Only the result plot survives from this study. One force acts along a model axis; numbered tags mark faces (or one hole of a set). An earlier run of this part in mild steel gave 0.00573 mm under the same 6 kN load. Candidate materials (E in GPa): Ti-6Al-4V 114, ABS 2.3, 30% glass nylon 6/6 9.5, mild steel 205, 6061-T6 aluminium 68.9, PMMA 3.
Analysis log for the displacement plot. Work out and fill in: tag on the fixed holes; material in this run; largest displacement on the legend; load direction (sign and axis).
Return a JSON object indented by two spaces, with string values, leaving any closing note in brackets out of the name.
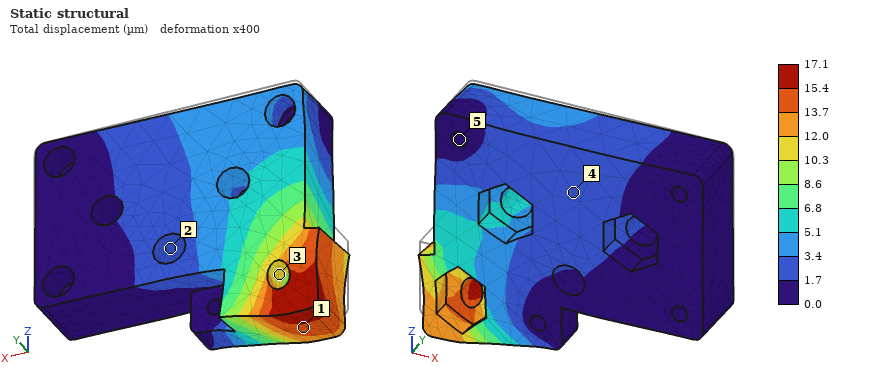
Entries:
{
  "tag on the fixed holes": "5",
  "material in this run": "6061-T6 aluminium",
  "largest displacement on the legend": "17.1 µm",
  "load direction": "-Z"
}
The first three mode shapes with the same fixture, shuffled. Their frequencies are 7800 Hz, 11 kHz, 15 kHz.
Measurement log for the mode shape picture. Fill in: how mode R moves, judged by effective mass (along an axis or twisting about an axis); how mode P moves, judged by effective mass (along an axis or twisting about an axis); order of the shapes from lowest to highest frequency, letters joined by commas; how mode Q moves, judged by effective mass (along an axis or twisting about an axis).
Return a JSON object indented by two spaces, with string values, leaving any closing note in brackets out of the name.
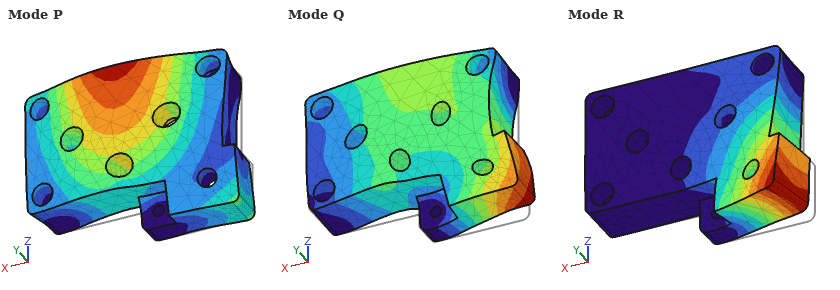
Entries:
{
  "how mode R moves, judged by effective mass": "along Y",
  "how mode P moves, judged by effective mass": "along Y",
  "order of the shapes from lowest to highest frequency, letters joined by commas": "R, P, Q",
  "how mode Q moves, judged by effective mass": "along Z"
}
